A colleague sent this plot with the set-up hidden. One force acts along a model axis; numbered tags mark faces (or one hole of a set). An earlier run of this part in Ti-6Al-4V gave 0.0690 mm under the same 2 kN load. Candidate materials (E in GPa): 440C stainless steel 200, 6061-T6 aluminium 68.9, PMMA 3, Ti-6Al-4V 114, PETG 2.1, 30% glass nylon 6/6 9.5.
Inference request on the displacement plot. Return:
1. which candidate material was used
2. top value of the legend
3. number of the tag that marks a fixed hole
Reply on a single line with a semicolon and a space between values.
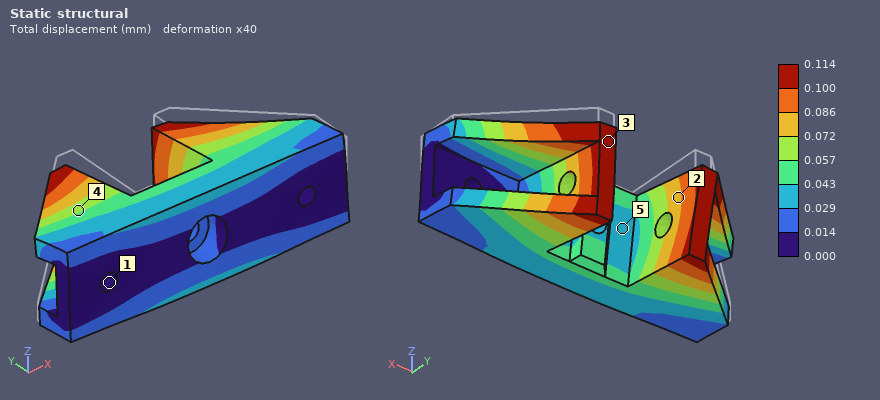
6061-T6 aluminium; 0.114 mm; 1
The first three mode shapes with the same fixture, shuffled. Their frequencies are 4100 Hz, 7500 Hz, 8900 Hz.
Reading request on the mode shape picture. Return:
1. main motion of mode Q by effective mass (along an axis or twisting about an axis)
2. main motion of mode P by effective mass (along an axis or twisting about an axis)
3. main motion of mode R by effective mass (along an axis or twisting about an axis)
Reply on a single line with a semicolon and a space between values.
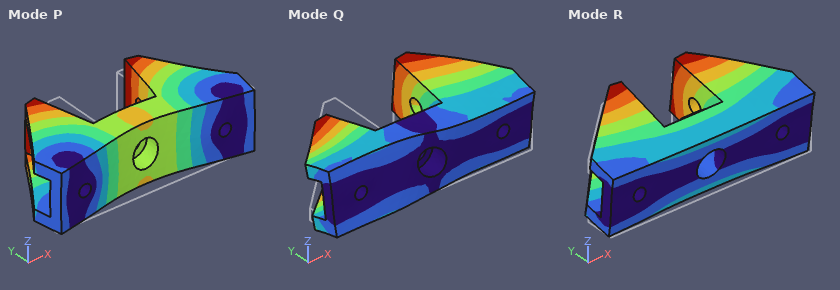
twisting about Y; along Y; along Z
